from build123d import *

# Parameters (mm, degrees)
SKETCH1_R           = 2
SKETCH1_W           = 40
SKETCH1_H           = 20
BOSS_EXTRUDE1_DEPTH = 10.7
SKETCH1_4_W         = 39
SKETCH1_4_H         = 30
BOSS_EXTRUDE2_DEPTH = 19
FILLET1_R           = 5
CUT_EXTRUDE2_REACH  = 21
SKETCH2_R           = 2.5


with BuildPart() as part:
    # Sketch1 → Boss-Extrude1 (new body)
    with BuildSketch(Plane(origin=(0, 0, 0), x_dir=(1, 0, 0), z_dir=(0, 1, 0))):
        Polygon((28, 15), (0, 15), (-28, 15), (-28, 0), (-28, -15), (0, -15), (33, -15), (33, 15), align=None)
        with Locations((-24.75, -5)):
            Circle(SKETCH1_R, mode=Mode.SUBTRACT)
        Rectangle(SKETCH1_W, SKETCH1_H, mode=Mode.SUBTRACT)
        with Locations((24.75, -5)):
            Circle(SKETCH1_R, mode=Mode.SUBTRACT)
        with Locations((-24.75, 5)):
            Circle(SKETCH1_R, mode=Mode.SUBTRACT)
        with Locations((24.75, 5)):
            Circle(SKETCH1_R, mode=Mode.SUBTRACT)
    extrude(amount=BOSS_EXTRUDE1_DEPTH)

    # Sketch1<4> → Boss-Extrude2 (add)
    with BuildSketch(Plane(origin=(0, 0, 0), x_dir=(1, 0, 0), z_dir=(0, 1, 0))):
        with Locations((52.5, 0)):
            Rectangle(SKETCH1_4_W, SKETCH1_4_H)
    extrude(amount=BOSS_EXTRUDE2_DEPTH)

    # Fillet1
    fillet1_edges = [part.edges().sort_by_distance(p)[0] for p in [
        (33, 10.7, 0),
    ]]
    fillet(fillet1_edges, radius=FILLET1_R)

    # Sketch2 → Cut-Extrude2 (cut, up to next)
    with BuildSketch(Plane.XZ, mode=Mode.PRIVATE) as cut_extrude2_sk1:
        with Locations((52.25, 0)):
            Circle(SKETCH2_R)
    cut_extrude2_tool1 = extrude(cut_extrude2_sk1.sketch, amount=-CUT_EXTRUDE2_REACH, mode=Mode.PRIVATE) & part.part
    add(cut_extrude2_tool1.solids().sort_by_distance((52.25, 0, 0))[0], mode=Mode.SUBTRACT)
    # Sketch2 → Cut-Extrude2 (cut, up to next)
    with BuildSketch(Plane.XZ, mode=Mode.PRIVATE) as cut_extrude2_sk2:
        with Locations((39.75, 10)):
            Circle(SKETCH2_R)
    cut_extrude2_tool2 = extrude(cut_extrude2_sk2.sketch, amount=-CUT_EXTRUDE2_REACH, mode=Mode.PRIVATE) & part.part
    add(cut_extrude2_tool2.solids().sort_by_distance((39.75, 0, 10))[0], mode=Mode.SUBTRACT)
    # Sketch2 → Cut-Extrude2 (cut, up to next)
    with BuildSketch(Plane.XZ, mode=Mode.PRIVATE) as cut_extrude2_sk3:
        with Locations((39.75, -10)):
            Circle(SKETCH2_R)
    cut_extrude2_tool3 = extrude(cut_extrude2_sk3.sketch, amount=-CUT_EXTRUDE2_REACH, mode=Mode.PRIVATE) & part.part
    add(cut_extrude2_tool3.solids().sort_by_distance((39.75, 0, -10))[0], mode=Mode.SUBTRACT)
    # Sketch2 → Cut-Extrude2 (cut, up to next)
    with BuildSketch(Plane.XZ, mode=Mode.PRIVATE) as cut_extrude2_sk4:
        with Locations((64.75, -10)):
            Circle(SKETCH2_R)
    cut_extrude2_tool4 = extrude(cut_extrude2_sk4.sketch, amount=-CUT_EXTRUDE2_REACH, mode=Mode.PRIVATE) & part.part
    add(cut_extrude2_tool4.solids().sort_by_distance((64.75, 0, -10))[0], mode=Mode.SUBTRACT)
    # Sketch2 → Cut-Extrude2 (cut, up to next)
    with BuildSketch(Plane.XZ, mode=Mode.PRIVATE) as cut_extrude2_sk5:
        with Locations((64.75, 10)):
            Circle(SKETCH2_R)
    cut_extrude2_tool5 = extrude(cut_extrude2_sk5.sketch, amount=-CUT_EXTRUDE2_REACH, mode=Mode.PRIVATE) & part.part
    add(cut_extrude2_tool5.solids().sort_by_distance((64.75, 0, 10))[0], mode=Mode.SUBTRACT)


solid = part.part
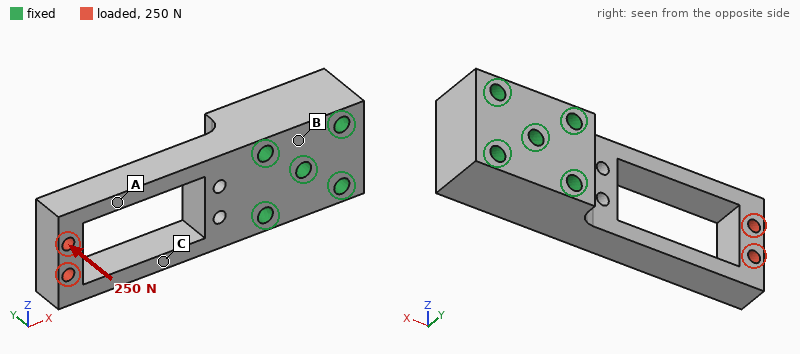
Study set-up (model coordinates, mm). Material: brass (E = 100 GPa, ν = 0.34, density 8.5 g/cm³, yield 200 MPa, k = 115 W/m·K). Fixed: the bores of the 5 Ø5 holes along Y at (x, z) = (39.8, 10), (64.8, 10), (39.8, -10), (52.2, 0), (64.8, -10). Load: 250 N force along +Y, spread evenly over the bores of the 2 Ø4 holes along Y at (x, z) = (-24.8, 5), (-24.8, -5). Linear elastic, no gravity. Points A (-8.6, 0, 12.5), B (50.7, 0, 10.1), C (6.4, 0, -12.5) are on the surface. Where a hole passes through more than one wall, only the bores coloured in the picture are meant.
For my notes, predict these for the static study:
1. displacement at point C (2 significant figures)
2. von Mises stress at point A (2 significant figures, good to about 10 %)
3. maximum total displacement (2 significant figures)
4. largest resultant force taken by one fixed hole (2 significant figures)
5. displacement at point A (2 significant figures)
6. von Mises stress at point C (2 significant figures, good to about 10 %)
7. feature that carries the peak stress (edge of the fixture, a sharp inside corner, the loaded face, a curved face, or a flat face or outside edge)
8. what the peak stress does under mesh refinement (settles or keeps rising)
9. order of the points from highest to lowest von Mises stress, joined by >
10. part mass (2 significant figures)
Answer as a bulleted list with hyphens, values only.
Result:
- 0.034 mm
- 21 MPa
- 0.14 mm
- 160 N
- 0.076 mm
- 41 MPa
- a sharp inside corner
- keeps rising
- C > A > B
- 260 g
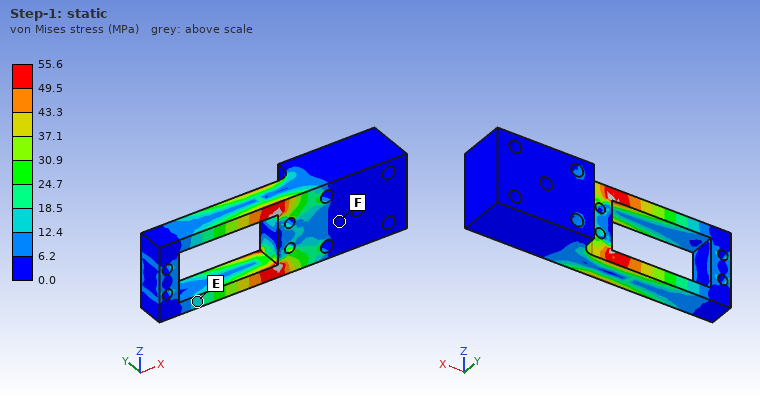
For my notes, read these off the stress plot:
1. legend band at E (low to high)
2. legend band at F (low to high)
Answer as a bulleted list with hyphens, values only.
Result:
- 12.4 to 18.5 MPa
- 0.0 to 6.2 MPa
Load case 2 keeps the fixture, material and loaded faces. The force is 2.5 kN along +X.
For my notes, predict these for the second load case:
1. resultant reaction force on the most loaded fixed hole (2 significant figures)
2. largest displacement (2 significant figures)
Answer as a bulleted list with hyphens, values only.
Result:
- 1.1 kN
- 32 µm
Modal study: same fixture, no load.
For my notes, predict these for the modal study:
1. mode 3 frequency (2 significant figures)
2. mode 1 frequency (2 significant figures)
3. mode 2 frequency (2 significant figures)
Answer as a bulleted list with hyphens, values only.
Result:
- 2900 Hz
- 1300 Hz
- 1400 Hz
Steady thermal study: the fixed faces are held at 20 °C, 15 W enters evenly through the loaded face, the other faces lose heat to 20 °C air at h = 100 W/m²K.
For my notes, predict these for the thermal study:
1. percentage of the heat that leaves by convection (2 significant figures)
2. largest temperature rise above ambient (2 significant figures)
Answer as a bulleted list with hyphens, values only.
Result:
- 57 %
- 39 K
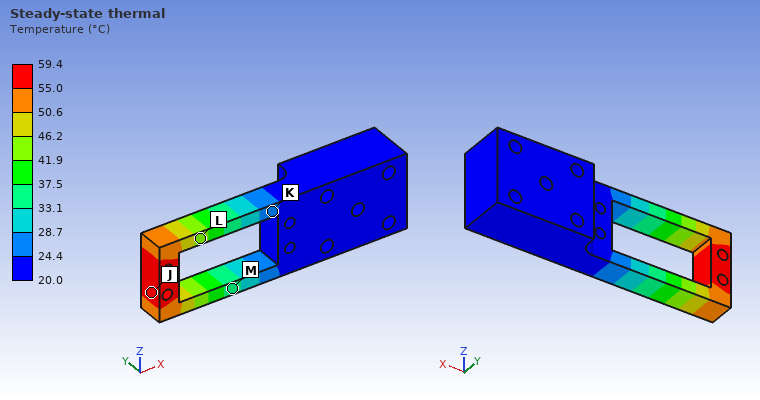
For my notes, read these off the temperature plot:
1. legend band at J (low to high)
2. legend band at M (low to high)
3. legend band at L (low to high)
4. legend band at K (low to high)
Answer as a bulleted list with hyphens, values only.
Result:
- 55.0 to 59.4 °C
- 33.1 to 37.5 °C
- 41.9 to 46.2 °C
- 24.4 to 28.7 °C
